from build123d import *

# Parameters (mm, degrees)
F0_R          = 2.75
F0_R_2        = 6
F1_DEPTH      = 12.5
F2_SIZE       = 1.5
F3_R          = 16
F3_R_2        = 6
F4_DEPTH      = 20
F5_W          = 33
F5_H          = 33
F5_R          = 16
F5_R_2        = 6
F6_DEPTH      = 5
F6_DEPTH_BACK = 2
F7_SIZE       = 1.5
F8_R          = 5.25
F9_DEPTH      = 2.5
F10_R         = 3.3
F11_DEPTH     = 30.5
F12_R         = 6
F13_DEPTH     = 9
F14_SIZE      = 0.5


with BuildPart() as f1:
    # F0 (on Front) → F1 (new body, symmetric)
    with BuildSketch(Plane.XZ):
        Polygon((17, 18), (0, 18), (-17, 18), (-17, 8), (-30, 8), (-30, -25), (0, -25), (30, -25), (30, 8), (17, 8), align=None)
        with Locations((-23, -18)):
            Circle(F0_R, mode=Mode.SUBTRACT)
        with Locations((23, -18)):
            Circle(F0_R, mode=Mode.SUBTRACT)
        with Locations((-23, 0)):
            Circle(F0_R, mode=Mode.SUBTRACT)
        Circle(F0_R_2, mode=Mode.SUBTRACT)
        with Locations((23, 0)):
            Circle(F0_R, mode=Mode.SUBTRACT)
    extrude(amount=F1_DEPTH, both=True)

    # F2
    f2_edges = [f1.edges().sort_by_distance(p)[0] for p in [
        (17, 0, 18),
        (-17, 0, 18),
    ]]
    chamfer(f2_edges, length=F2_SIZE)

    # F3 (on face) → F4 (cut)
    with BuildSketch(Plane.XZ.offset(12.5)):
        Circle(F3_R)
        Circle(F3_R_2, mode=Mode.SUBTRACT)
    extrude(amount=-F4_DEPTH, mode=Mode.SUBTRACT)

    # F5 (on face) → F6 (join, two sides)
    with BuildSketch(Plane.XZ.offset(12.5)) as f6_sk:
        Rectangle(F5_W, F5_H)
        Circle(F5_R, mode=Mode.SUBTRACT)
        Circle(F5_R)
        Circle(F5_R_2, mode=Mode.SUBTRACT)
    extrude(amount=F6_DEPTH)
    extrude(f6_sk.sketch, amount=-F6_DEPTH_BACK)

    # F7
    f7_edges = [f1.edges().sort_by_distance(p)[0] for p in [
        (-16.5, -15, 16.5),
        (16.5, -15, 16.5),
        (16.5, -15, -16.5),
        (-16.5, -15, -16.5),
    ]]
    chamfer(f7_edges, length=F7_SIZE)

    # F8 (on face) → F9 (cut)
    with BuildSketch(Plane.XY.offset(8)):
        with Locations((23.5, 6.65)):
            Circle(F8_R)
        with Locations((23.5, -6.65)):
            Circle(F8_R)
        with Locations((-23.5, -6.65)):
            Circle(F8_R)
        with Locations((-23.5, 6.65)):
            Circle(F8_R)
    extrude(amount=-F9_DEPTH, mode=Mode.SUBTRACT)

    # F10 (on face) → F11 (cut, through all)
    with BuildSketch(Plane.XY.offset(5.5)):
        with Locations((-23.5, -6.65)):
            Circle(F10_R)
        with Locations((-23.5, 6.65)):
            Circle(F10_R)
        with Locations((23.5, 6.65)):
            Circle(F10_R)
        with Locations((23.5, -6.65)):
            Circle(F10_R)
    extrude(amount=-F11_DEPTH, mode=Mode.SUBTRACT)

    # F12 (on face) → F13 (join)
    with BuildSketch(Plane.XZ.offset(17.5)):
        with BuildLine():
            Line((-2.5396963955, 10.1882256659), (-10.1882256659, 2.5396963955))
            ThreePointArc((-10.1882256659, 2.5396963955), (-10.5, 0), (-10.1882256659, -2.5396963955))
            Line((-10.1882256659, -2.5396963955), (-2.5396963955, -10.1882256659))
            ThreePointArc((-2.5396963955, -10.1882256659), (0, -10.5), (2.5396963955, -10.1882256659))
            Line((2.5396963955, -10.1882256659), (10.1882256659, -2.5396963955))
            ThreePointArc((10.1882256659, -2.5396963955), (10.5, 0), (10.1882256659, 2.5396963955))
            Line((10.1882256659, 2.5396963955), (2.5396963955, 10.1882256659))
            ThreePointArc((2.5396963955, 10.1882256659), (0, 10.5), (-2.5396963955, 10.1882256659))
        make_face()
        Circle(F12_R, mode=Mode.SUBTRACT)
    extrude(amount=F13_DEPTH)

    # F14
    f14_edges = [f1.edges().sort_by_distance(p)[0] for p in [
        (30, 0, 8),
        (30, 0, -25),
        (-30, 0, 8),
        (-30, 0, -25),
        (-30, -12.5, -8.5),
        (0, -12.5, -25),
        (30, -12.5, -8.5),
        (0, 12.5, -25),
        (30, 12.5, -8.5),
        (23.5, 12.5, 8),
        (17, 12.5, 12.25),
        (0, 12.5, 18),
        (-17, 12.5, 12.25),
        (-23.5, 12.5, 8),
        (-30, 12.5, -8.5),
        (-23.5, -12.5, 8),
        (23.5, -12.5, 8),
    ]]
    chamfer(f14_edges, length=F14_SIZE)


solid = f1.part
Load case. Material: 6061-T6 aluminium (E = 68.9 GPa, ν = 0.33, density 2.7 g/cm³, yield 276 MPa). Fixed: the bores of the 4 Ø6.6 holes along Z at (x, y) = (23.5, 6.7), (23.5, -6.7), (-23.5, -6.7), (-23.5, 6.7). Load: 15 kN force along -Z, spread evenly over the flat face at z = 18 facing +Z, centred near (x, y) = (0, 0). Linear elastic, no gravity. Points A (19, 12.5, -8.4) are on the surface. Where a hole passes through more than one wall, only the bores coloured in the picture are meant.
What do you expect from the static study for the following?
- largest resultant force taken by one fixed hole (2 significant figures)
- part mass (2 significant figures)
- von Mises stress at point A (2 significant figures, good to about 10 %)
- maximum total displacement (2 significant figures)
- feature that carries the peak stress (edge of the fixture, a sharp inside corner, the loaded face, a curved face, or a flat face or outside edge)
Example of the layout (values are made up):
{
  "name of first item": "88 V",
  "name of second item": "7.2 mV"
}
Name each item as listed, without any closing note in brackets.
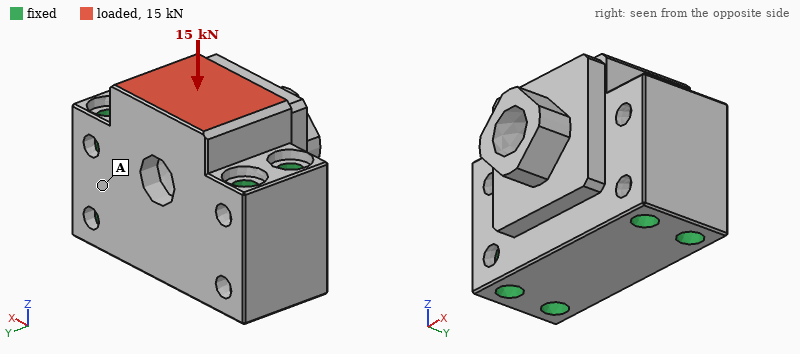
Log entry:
{
  "largest resultant force taken by one fixed hole": "4.3 kN",
  "part mass": "120 g",
  "von Mises stress at point A": "23 MPa",
  "maximum total displacement": "60 µm",
  "feature that carries the peak stress": "the loaded face"
}
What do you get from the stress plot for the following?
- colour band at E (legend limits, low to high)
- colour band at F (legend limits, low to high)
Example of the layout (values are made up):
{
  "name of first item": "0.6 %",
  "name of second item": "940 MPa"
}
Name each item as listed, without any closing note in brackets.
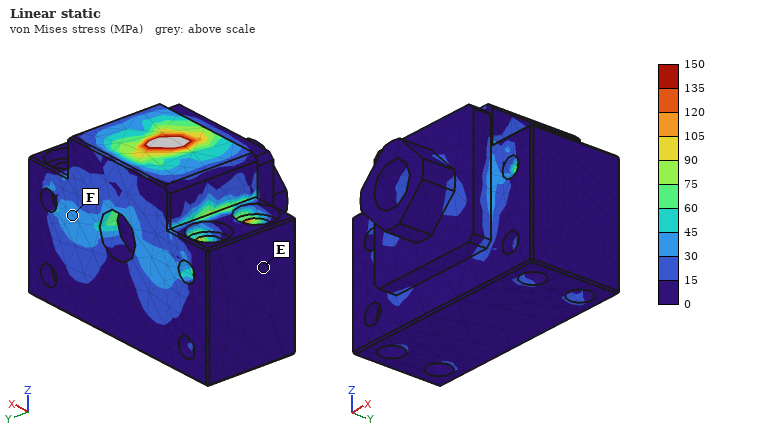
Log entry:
{
  "colour band at E": "0 to 15 MPa",
  "colour band at F": "30 to 45 MPa"
}
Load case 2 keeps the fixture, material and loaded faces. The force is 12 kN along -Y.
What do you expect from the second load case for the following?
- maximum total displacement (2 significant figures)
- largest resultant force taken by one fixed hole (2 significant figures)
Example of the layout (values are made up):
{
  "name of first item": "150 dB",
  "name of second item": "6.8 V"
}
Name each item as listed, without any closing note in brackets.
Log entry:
{
  "maximum total displacement": "67 µm",
  "largest resultant force taken by one fixed hole": "5.3 kN"
}
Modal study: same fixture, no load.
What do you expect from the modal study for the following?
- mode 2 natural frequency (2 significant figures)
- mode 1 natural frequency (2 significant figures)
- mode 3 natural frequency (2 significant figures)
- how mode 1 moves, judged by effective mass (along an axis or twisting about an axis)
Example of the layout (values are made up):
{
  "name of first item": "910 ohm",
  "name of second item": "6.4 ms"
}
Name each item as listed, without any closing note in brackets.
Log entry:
{
  "mode 2 natural frequency": "26 kHz",
  "mode 1 natural frequency": "17 kHz",
  "mode 3 natural frequency": "26 kHz",
  "how mode 1 moves, judged by effective mass": "along Y"
}
